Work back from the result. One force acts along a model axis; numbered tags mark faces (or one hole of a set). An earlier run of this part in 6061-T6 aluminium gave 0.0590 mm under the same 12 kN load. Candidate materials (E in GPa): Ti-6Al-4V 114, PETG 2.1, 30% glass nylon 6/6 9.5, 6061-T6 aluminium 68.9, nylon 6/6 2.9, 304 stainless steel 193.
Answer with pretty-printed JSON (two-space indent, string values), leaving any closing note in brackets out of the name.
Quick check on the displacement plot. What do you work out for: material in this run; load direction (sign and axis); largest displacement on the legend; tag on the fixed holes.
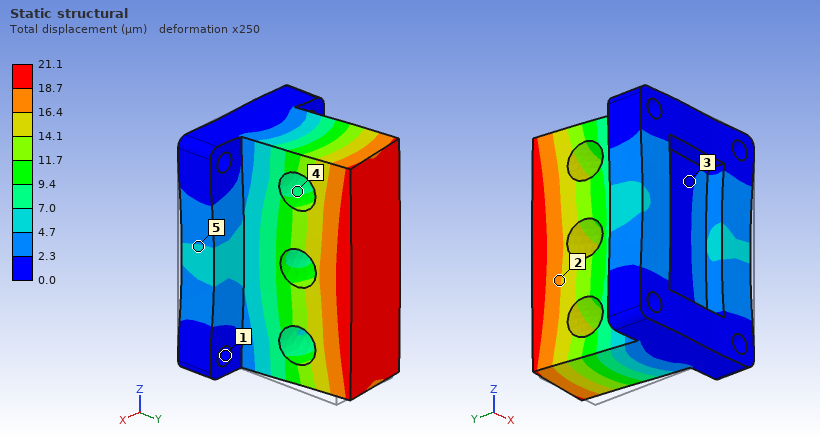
{
  "material in this run": "304 stainless steel",
  "load direction": "-X",
  "largest displacement on the legend": "21.1 µm",
  "tag on the fixed holes": "1"
}
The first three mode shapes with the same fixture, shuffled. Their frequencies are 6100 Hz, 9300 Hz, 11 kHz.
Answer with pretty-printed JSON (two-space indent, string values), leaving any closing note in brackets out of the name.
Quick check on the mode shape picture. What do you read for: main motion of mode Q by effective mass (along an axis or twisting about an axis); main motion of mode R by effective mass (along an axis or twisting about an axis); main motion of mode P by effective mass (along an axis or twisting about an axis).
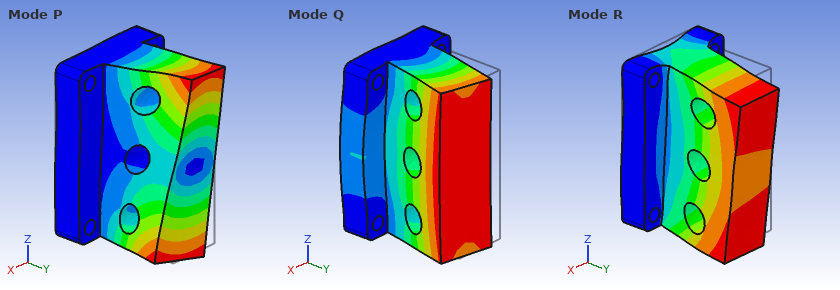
{
  "main motion of mode Q by effective mass": "along X",
  "main motion of mode R by effective mass": "along Z",
  "main motion of mode P by effective mass": "twisting about Y"
}
